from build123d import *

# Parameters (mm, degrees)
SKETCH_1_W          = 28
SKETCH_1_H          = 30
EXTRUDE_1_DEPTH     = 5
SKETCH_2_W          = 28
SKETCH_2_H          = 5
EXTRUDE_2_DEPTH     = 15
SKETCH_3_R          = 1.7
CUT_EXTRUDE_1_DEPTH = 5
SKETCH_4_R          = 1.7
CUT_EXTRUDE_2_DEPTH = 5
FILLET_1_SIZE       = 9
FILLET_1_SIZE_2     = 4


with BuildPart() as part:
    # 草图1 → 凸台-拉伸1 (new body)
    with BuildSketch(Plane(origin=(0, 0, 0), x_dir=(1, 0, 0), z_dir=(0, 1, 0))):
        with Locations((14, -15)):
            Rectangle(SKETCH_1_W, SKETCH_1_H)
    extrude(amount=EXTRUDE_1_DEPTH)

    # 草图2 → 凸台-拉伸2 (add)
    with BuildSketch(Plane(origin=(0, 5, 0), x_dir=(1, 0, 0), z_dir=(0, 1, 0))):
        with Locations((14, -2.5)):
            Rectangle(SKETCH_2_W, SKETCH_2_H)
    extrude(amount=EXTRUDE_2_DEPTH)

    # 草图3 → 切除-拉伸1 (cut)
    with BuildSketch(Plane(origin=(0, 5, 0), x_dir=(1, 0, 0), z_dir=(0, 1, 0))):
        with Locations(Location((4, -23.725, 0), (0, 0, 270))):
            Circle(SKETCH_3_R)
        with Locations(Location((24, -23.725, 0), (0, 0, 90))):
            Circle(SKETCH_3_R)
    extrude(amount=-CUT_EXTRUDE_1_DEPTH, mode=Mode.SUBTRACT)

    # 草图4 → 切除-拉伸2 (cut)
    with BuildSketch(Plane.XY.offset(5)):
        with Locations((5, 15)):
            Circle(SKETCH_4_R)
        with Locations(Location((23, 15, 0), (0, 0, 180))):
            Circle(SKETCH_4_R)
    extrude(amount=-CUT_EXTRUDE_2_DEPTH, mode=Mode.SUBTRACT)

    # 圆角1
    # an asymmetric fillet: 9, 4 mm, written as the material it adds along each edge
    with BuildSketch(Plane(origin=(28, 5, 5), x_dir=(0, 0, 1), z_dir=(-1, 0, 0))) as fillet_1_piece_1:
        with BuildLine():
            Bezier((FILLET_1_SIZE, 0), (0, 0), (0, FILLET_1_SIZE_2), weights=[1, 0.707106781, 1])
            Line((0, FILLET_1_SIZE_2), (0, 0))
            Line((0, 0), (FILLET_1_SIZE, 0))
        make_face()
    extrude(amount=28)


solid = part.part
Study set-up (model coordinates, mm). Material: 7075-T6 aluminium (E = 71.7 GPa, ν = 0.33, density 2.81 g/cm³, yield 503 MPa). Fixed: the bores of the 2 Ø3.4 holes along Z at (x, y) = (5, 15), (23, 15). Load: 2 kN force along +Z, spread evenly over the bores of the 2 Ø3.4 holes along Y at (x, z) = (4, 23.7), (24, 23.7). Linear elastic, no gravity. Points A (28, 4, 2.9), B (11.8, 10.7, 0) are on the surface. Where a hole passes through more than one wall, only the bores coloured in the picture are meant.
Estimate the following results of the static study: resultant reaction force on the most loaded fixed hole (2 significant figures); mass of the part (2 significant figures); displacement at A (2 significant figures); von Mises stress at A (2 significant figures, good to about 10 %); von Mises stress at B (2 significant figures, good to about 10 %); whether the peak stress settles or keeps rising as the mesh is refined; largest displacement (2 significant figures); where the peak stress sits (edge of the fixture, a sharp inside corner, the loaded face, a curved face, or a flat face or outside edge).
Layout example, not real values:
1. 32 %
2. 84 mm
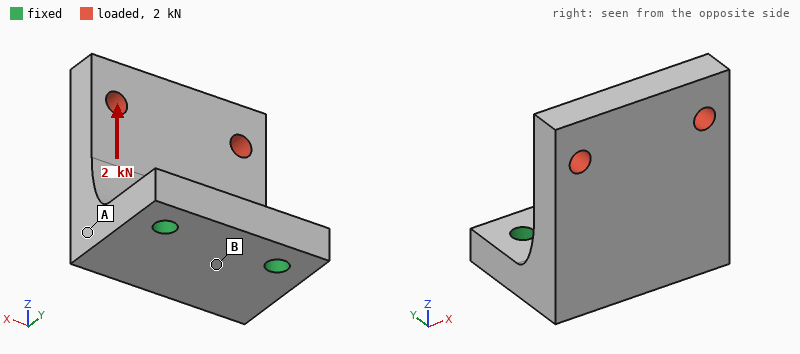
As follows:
1. 1.0 kN
2. 18 g
3. 0.058 mm
4. 37 MPa
5. 89 MPa
6. keeps rising
7. 0.22 mm
8. edge of the fixture
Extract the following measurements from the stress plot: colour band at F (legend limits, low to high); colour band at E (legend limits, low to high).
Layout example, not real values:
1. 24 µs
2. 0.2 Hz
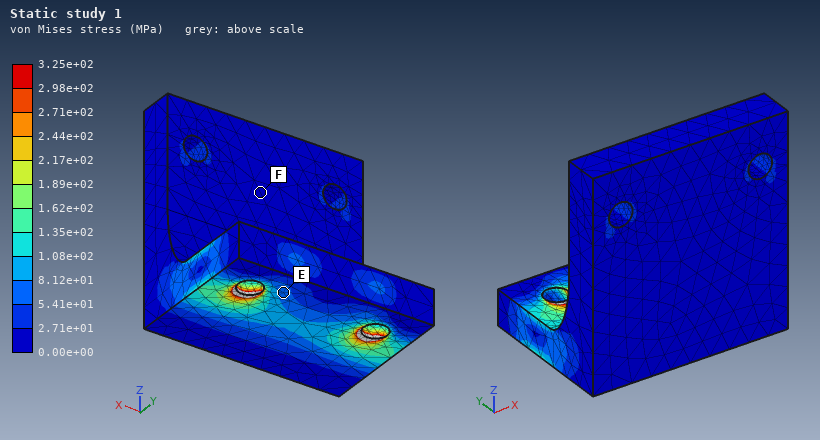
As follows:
1. 0.00e+00 to 2.71e+01 MPa
2. 5.41e+01 to 8.12e+01 MPa
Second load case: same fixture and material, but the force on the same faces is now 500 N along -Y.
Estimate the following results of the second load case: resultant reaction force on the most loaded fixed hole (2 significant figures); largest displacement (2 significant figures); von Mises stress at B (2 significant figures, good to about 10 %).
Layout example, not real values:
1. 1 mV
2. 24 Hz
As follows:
1. 270 N
2. 0.20 mm
3. 63 MPa
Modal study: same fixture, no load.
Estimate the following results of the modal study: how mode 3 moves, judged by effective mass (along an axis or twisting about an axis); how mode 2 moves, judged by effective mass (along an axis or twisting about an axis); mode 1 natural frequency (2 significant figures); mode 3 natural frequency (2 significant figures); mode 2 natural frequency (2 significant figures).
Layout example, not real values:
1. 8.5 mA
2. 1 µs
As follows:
1. along Z
2. along X
3. 3700 Hz
4. 13 kHz
5. 7500 Hz
